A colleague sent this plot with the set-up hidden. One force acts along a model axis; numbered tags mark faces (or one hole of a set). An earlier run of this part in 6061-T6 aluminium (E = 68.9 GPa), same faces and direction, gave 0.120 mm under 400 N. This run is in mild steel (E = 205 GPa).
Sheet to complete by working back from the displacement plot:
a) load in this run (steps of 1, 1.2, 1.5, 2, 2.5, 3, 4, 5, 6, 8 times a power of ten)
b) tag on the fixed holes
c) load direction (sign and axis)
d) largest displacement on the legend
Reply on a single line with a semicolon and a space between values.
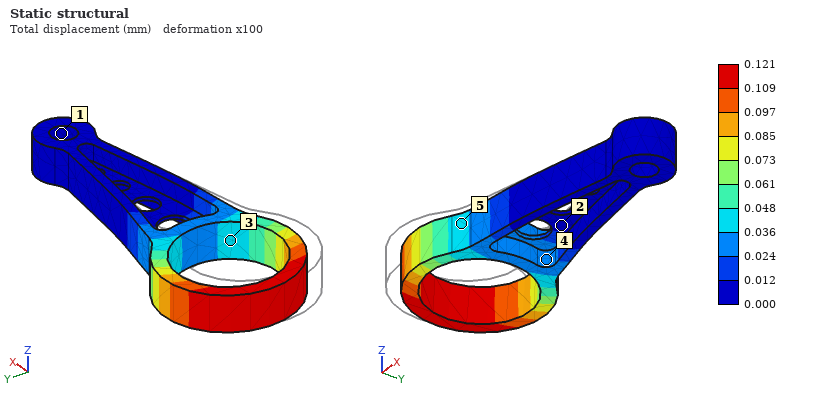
1.2 kN; 1; +Y; 0.121 mm
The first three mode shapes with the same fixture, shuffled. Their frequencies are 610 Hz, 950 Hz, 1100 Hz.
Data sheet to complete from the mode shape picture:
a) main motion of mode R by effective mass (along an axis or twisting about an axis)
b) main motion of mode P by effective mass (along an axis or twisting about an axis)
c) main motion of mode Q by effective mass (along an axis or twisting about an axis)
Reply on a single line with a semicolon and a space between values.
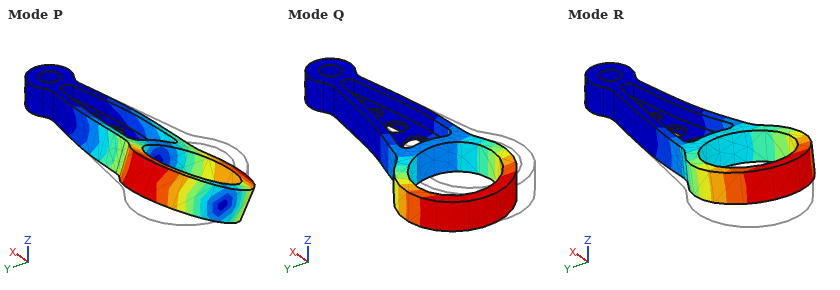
along Z; twisting about X; along Y
